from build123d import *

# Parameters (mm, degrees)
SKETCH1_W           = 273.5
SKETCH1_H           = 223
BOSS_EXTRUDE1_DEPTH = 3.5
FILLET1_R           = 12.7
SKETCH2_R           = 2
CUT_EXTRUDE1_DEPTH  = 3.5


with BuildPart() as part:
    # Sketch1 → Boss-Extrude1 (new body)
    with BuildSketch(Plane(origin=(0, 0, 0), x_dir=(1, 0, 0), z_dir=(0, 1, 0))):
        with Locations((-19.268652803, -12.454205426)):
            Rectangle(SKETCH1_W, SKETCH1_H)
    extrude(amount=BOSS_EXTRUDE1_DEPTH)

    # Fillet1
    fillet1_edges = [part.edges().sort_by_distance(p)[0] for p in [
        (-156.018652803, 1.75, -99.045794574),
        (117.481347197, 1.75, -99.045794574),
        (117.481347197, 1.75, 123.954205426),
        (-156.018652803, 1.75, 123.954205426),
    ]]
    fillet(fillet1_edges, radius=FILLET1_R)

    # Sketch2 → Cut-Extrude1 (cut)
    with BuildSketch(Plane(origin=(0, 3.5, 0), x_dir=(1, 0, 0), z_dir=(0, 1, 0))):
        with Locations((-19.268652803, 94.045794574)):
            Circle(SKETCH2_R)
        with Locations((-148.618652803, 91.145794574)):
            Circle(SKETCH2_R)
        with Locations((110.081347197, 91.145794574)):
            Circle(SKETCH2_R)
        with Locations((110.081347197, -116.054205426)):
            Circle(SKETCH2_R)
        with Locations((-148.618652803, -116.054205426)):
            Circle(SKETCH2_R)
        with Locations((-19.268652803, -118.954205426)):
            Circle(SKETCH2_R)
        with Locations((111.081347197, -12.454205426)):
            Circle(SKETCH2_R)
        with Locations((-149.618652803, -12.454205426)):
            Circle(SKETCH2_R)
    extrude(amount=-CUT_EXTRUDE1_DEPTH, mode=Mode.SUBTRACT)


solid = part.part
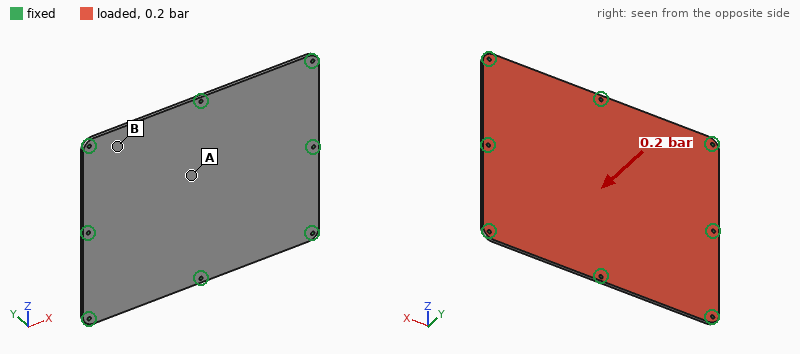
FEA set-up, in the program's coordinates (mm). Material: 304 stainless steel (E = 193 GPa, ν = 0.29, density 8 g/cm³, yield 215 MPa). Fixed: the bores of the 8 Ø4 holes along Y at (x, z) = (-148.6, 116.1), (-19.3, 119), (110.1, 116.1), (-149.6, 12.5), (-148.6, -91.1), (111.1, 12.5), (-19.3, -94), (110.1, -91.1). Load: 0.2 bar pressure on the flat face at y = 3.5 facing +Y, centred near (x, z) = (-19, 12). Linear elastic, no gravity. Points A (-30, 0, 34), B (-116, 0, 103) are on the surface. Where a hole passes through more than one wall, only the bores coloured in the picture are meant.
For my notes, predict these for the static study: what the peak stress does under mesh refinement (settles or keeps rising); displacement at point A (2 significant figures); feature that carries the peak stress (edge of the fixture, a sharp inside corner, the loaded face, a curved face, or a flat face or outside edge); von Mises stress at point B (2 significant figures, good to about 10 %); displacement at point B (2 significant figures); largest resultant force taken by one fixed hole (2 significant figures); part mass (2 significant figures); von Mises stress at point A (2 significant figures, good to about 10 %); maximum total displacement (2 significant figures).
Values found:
keeps rising
0.16 mm
edge of the fixture
5.8 MPa
0.031 mm
260 N
1.7 kg
15 MPa
0.17 mm
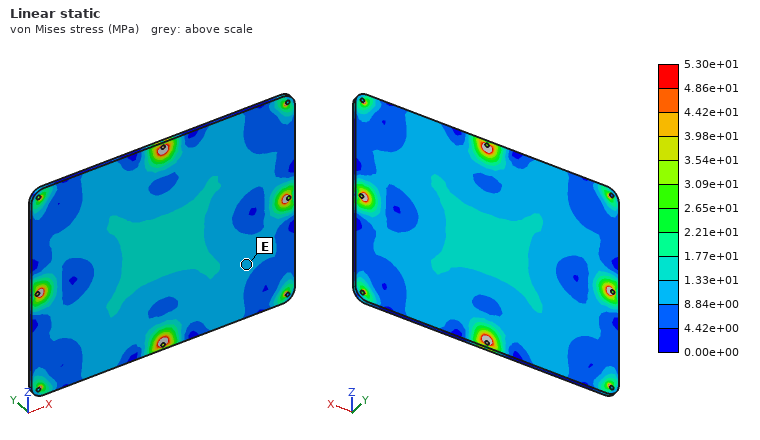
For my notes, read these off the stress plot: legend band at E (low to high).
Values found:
8.84e+00 to 1.33e+01 MPa
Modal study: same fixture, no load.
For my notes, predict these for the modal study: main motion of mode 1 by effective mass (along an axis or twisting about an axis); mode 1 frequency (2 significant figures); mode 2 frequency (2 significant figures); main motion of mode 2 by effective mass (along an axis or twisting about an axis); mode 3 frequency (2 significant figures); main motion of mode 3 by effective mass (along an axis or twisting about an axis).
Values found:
along Y
410 Hz
670 Hz
twisting about Z
810 Hz
twisting about X
